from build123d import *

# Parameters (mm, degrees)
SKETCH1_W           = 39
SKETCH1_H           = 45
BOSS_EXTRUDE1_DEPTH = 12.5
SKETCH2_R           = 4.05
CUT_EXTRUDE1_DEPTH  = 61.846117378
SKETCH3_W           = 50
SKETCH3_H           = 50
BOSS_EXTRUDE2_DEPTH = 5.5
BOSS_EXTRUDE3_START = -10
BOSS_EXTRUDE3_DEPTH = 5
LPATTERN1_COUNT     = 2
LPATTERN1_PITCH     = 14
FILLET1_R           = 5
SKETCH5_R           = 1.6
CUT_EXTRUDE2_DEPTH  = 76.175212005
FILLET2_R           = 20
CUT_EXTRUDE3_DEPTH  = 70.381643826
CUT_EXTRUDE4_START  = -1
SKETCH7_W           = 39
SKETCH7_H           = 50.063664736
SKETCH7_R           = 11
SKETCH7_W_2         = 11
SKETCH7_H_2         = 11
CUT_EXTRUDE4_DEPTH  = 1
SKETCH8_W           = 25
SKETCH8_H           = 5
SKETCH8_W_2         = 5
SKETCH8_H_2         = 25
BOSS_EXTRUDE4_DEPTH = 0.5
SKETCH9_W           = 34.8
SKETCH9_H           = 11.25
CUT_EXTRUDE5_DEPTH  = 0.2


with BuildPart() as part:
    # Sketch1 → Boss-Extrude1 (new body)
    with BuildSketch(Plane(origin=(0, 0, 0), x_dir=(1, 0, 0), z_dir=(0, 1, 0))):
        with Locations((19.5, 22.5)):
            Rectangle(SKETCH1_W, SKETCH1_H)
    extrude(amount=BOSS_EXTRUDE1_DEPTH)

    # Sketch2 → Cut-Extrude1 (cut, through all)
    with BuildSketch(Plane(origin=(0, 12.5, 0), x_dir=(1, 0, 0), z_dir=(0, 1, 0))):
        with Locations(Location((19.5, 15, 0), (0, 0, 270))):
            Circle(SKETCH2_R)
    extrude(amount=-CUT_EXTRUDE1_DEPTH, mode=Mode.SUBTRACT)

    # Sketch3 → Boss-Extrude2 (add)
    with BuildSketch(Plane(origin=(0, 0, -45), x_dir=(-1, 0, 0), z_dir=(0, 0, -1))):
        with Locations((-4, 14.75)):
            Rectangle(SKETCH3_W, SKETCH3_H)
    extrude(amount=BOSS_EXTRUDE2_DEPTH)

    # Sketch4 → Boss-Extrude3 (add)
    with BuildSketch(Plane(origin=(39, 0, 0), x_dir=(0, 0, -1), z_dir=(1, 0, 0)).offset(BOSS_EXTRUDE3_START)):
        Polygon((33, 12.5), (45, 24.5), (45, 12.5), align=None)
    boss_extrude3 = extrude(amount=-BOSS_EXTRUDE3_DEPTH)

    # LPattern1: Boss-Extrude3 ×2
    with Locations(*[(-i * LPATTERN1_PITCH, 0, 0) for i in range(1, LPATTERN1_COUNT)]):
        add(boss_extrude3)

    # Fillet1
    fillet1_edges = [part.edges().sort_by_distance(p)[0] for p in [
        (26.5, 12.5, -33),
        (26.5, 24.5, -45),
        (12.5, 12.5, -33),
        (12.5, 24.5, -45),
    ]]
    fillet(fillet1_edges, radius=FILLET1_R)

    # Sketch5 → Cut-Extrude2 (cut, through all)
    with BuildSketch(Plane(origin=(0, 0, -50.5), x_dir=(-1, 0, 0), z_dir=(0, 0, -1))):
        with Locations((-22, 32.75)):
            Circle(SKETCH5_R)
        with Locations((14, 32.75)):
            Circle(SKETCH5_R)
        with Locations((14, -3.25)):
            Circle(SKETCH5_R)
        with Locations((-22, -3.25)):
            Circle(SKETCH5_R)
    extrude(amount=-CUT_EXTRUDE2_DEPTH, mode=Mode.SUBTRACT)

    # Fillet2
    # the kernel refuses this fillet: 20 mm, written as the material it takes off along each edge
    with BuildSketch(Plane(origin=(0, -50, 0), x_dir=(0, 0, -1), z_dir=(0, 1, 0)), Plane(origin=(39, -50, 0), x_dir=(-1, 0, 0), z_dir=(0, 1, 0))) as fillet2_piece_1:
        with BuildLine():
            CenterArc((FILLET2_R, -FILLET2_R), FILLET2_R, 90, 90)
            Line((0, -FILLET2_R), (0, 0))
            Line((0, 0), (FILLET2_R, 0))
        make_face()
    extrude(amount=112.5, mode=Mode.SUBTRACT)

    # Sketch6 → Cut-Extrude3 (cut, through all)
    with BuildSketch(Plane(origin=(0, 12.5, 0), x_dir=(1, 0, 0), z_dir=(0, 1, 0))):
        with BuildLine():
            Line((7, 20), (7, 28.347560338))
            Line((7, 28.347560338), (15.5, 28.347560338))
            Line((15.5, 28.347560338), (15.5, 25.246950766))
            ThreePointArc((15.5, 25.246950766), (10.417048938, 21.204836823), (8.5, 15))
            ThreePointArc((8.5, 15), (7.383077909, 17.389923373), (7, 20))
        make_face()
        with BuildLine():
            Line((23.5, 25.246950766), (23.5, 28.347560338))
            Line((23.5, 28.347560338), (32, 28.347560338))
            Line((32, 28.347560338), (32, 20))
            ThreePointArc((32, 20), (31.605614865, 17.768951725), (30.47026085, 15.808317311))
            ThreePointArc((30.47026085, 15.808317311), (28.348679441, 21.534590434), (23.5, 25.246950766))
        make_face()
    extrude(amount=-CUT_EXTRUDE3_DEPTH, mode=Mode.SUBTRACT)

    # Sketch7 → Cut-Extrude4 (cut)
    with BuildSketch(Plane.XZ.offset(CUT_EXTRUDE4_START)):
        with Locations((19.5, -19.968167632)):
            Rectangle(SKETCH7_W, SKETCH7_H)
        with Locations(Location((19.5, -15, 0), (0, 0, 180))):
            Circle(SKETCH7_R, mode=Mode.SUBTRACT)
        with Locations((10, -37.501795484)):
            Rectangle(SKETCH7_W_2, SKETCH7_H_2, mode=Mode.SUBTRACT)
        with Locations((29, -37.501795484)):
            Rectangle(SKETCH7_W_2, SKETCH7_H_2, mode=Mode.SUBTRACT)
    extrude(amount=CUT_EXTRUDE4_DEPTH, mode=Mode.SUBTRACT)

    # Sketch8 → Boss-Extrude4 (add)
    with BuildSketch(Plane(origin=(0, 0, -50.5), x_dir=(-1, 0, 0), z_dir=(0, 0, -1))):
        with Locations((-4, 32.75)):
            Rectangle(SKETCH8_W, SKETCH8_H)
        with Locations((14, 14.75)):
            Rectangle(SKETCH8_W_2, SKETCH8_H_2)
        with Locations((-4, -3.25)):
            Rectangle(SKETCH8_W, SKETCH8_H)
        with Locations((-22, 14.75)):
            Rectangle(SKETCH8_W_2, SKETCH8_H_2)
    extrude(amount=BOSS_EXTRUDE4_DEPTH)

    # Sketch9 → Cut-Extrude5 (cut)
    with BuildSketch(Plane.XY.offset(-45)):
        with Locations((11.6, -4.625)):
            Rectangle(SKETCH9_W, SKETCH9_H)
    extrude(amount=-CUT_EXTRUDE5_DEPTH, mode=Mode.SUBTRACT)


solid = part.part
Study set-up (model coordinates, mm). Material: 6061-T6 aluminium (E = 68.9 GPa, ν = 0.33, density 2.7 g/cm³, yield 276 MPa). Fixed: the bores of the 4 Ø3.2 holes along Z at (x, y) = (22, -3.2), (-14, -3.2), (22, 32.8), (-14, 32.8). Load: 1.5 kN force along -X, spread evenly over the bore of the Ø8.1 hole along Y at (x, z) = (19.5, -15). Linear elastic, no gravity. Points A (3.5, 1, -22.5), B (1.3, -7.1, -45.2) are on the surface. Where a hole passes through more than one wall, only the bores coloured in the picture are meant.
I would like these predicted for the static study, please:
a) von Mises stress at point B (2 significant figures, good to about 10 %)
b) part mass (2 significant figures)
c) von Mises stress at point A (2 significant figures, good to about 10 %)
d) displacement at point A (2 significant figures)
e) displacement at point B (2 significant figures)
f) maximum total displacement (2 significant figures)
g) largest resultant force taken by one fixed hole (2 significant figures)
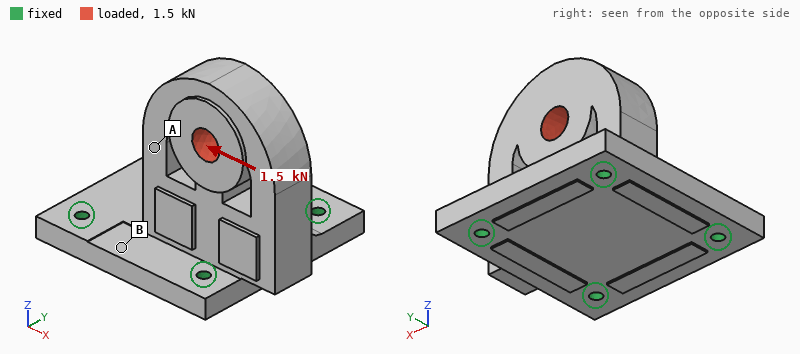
34 MPa
85 g
13 MPa
0.062 mm
0.016 mm
0.11 mm
1.2 kN
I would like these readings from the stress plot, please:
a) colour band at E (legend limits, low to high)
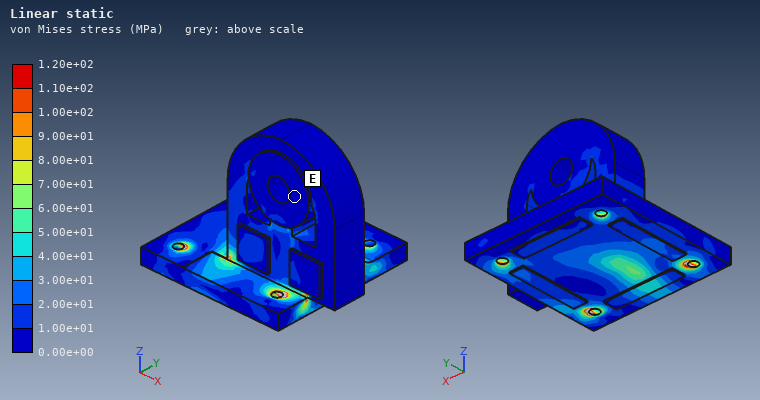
0.00e+00 to 1.00e+01 MPa
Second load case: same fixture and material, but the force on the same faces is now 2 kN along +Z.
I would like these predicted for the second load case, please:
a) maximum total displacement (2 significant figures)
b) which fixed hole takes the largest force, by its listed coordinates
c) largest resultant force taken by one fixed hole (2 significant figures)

17 µm
(22, -3.2)
1.4 kN
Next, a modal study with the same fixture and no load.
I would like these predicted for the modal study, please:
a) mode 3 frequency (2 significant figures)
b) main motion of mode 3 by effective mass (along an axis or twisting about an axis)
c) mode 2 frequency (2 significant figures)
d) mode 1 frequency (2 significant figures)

9500 Hz
along Z
4000 Hz
3800 Hz
